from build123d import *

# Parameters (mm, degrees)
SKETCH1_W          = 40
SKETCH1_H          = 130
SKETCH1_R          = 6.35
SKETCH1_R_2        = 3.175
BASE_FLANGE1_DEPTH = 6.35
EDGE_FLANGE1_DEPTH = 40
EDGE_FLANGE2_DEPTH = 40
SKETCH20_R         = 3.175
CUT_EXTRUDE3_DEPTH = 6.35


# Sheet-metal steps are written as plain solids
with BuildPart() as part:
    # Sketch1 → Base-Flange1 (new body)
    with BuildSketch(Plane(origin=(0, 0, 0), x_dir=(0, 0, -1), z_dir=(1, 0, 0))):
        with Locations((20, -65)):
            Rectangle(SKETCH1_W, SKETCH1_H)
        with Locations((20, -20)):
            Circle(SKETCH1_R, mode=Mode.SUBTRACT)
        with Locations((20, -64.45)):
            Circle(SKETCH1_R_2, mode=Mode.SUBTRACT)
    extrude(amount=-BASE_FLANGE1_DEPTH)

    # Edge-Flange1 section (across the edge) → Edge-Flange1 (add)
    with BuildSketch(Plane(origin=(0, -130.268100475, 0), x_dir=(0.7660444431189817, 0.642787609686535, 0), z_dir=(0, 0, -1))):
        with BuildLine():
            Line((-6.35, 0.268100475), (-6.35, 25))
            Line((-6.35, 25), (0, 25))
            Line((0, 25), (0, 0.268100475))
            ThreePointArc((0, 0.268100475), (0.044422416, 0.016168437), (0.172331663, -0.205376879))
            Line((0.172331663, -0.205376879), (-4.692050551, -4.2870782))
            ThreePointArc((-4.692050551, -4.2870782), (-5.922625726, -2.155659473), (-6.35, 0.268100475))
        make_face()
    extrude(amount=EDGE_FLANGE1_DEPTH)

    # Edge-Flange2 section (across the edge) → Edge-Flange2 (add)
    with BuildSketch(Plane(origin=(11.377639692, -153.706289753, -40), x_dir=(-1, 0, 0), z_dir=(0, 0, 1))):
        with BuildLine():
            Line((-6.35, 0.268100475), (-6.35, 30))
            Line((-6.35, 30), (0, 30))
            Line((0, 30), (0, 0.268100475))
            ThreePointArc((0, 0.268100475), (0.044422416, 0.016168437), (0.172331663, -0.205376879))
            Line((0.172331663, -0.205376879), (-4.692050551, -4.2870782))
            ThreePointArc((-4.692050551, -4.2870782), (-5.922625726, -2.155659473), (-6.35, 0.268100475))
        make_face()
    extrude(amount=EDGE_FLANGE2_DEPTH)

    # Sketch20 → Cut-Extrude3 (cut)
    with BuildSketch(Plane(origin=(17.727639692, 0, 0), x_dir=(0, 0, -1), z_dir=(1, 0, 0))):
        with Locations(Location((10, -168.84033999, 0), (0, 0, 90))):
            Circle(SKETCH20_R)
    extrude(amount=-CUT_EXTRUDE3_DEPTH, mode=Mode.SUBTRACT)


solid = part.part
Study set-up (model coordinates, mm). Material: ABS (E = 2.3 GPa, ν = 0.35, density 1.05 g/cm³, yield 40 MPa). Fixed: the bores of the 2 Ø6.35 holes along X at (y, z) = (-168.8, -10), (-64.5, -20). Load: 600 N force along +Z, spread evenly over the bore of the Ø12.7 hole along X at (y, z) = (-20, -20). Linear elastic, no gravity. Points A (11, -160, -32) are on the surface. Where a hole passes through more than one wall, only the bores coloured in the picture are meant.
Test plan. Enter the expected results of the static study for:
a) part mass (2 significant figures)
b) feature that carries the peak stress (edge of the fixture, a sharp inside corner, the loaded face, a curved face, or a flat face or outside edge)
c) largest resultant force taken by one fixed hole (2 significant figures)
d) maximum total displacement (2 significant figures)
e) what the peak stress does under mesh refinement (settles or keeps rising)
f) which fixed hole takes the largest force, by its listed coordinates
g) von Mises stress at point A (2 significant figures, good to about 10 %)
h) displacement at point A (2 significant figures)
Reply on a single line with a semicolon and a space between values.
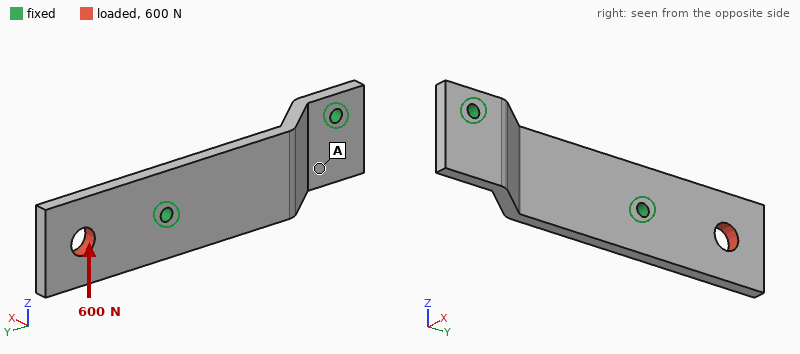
49 g; edge of the fixture; 790 N; 1.5 mm; keeps rising; (-64.5, -20); 4.3 MPa; 0.26 mm
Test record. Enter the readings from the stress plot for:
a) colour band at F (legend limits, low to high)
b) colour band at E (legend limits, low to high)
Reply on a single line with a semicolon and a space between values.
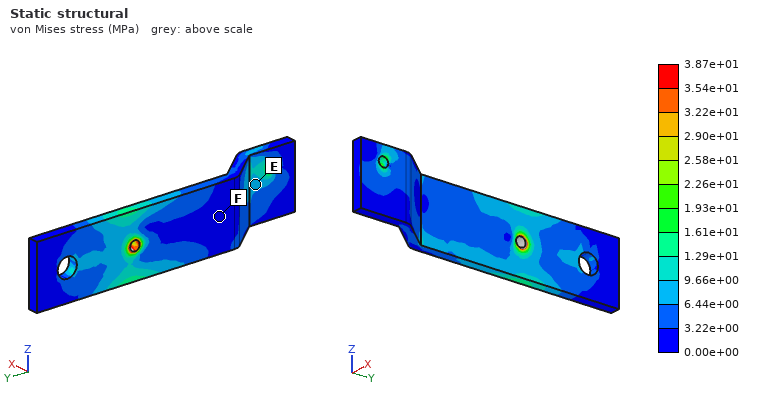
0.00e+00 to 3.22e+00 MPa; 6.44e+00 to 9.66e+00 MPa
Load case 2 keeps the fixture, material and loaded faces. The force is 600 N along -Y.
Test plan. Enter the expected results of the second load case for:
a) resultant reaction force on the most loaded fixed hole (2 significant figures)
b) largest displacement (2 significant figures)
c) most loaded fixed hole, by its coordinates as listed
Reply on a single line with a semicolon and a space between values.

590 N; 81 µm; (-64.5, -20)
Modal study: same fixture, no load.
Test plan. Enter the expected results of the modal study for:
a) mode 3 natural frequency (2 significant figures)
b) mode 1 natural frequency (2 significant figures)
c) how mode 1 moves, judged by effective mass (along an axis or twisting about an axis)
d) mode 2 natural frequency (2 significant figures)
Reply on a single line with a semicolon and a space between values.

1000 Hz; 370 Hz; along X; 820 Hz
